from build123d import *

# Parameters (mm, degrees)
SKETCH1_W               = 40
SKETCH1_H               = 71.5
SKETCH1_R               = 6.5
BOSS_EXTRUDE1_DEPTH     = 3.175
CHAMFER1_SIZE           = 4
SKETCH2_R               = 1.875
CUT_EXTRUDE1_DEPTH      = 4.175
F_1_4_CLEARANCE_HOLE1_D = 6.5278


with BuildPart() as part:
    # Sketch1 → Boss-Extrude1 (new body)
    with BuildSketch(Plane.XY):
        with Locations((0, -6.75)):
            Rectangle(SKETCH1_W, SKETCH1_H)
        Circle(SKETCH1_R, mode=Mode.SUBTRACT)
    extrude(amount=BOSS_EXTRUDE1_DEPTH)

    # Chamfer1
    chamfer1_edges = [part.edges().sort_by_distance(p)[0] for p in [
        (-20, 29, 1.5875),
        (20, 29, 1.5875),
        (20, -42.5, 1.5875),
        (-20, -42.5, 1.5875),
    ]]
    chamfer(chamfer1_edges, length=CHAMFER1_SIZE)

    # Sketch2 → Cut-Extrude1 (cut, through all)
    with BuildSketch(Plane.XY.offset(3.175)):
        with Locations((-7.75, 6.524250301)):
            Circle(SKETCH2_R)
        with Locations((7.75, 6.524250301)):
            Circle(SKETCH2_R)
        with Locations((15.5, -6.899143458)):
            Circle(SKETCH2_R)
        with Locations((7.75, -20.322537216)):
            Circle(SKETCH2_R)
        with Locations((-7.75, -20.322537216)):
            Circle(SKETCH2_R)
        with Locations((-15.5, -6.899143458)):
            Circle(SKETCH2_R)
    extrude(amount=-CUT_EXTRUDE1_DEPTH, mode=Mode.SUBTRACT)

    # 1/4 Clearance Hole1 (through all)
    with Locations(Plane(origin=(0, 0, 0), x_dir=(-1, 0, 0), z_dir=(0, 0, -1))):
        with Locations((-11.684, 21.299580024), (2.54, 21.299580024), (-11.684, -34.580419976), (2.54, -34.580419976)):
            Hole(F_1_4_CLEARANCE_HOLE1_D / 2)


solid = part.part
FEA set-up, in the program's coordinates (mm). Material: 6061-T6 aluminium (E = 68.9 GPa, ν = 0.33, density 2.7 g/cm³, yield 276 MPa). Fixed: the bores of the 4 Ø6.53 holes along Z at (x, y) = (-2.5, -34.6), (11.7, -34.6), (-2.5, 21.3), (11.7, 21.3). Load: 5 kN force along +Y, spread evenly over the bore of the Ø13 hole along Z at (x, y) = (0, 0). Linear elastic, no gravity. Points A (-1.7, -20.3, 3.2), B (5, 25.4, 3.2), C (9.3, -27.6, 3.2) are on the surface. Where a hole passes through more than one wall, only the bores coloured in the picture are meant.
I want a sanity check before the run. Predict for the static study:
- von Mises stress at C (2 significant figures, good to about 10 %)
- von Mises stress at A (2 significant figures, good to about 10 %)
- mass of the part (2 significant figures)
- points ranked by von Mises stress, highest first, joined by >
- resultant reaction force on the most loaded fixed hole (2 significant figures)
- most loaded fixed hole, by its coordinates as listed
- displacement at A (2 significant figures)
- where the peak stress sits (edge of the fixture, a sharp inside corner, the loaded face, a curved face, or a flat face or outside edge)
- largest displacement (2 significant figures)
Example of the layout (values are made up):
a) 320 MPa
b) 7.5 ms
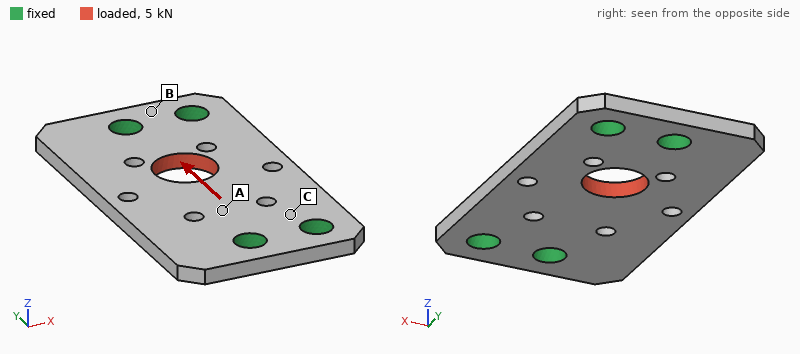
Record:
a) 20 MPa
b) 32 MPa
c) 21 g
d) A > C > B
e) 1.8 kN
f) (-2.5, 21.3)
g) 5.6 µm
h) a curved face
i) 15 µm
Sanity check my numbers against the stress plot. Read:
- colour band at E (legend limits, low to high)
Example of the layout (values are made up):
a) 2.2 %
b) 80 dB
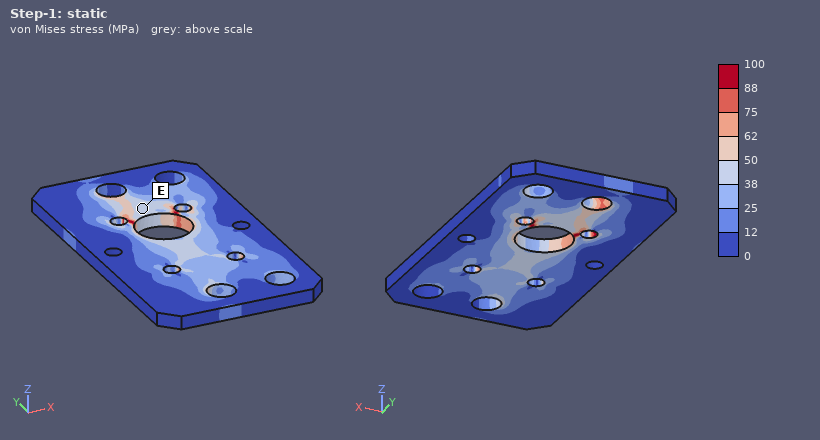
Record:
a) 38 to 50 MPa
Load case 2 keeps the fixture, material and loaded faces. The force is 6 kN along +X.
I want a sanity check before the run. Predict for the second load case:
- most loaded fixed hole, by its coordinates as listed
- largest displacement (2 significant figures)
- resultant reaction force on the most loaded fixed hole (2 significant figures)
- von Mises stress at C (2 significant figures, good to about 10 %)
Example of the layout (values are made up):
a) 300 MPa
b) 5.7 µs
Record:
a) (-2.5, 21.3)
b) 38 µm
c) 2.3 kN
d) 57 MPa
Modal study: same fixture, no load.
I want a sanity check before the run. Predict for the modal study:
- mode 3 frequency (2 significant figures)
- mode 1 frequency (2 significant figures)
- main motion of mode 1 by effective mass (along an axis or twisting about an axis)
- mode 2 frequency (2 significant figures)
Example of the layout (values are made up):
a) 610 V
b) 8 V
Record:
a) 10 kHz
b) 5200 Hz
c) along Z
d) 6800 Hz
